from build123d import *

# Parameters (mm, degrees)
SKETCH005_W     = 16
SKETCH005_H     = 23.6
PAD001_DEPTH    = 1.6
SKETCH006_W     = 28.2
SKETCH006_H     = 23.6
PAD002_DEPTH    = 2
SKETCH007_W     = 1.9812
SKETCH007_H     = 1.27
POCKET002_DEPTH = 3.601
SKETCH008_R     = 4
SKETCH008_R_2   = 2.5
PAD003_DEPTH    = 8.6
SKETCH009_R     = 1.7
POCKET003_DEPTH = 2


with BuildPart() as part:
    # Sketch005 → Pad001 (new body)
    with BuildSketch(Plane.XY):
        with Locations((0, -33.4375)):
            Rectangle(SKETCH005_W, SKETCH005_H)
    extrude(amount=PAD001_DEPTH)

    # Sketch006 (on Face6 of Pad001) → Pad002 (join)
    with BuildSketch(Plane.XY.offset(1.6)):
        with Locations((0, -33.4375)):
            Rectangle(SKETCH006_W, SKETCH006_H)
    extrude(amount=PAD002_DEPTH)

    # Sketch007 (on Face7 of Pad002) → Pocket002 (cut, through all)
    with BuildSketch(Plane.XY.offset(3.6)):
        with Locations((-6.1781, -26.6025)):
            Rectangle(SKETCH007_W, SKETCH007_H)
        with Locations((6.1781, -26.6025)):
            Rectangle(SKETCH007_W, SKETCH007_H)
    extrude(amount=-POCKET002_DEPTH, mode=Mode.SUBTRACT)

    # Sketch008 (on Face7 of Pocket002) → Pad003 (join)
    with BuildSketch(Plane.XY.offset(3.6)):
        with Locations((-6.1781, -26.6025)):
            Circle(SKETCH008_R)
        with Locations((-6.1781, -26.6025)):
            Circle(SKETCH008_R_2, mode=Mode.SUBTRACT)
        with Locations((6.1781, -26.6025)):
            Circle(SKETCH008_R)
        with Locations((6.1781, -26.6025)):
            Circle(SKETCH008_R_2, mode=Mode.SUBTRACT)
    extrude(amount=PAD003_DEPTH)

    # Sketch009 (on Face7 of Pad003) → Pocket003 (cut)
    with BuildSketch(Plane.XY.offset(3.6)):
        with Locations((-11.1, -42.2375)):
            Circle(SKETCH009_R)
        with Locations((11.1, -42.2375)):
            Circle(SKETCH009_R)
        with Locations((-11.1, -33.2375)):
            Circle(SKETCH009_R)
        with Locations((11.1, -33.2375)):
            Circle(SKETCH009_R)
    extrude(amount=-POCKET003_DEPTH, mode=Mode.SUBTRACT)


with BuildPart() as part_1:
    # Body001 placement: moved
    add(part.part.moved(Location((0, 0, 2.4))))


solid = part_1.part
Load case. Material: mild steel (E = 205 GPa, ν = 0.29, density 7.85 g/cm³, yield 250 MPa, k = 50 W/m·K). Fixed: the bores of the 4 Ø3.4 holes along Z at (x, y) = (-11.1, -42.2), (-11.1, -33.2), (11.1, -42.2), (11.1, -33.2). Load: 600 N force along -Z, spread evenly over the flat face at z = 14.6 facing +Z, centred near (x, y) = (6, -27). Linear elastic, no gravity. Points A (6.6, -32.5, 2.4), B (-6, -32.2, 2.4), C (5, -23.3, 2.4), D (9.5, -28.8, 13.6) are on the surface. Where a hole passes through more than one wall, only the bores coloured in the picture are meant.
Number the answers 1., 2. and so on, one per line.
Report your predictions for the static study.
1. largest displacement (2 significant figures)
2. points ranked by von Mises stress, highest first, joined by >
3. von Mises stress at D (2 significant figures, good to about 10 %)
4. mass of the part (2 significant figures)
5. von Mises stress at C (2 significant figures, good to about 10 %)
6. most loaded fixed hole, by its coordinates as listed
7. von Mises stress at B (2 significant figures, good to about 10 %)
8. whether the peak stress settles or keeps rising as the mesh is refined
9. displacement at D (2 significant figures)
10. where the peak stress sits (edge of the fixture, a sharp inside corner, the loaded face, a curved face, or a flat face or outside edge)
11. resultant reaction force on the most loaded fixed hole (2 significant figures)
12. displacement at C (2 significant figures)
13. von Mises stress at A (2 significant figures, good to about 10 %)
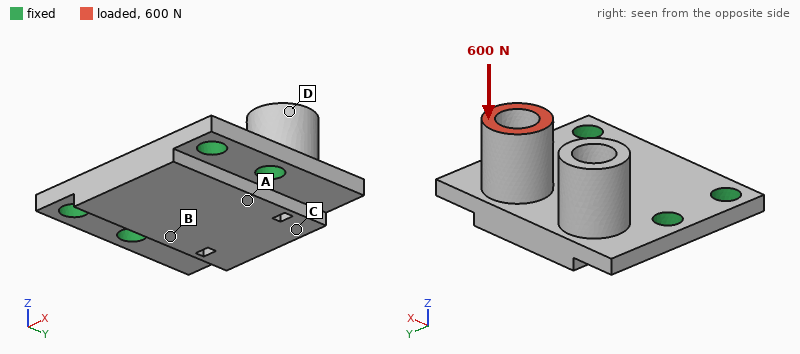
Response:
1. 27 µm
2. A > B > C > D
3. 18 MPa
4. 19 g
5. 39 MPa
6. (11.1, -33.2)
7. 57 MPa
8. keeps rising
9. 18 µm
10. edge of the fixture
11. 630 N
12. 18 µm
13. 87 MPa
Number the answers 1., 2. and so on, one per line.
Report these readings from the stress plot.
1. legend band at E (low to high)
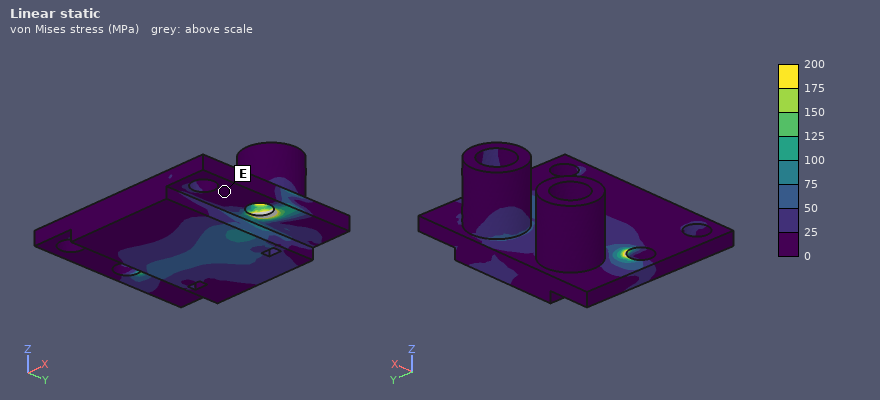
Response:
1. 0 to 25 MPa
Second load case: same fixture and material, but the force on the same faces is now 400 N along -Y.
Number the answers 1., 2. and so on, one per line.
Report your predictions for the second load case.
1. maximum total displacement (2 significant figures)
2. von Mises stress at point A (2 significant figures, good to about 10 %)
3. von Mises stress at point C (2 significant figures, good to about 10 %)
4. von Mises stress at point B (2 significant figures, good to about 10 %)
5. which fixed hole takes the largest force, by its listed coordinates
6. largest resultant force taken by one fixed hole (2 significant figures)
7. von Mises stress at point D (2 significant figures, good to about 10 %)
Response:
1. 39 µm
2. 99 MPa
3. 57 MPa
4. 64 MPa
5. (11.1, -33.2)
6. 420 N
7. 30 MPa
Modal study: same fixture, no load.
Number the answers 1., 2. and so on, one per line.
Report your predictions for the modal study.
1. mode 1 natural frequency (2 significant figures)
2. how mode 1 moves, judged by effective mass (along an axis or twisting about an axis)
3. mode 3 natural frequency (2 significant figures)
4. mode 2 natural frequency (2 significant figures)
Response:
1. 9500 Hz
2. along Z
3. 22 kHz
4. 18 kHz
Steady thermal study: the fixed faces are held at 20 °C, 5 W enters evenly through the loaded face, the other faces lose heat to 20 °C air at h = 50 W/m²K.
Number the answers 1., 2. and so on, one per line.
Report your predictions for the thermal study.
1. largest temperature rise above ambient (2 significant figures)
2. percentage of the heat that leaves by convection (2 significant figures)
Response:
1. 40 K
2. 18 %
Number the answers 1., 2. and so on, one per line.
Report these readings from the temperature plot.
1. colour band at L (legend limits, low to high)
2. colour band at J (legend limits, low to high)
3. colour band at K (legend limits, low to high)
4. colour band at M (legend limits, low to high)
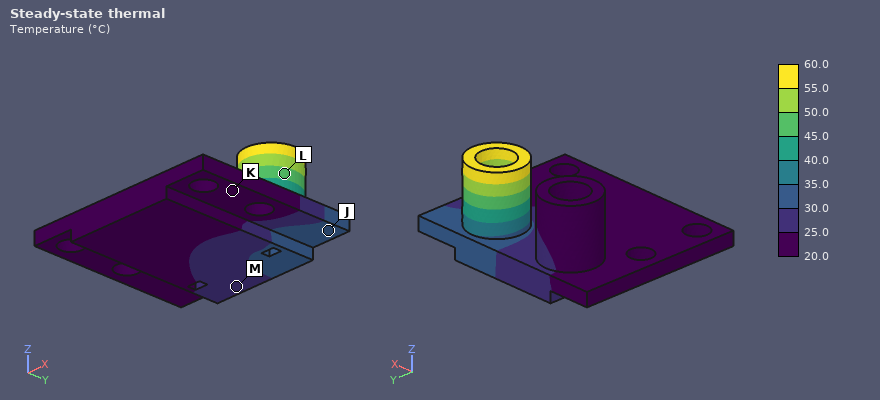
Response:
1. 45.0 to 50.0 °C
2. 30.0 to 35.0 °C
3. 20.0 to 25.0 °C
4. 25.0 to 30.0 °C
